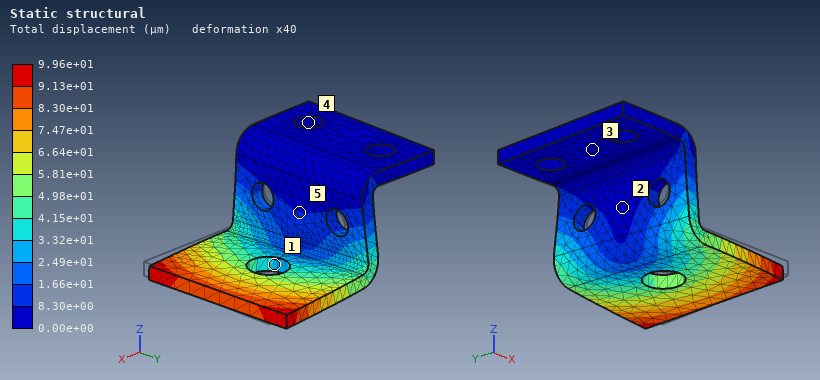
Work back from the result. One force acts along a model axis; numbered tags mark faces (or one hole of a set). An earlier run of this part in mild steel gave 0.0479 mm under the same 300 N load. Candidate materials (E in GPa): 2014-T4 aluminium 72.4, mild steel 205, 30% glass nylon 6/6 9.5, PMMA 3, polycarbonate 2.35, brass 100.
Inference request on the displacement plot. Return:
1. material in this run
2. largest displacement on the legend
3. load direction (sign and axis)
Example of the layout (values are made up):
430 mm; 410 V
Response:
brass; 9.96e+01 µm; +Y
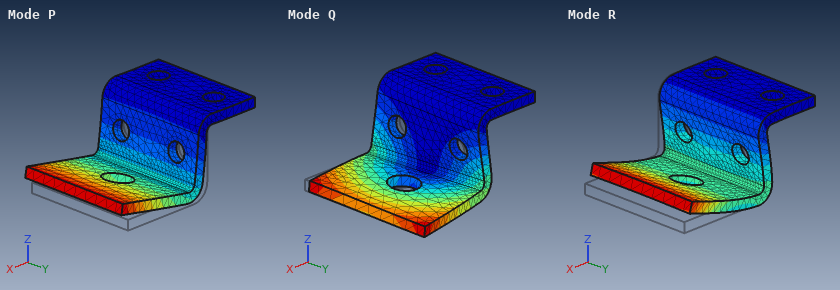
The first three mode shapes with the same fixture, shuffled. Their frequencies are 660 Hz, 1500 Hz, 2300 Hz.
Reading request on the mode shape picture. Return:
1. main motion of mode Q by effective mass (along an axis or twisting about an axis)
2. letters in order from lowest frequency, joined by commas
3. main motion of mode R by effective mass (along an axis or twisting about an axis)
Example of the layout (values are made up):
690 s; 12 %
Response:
along Y; P, Q, R; along X
